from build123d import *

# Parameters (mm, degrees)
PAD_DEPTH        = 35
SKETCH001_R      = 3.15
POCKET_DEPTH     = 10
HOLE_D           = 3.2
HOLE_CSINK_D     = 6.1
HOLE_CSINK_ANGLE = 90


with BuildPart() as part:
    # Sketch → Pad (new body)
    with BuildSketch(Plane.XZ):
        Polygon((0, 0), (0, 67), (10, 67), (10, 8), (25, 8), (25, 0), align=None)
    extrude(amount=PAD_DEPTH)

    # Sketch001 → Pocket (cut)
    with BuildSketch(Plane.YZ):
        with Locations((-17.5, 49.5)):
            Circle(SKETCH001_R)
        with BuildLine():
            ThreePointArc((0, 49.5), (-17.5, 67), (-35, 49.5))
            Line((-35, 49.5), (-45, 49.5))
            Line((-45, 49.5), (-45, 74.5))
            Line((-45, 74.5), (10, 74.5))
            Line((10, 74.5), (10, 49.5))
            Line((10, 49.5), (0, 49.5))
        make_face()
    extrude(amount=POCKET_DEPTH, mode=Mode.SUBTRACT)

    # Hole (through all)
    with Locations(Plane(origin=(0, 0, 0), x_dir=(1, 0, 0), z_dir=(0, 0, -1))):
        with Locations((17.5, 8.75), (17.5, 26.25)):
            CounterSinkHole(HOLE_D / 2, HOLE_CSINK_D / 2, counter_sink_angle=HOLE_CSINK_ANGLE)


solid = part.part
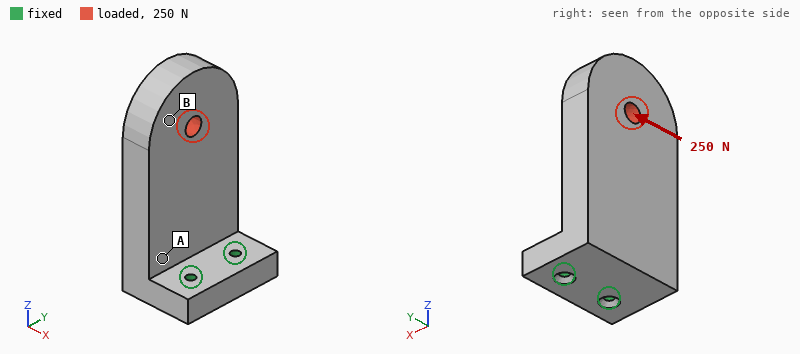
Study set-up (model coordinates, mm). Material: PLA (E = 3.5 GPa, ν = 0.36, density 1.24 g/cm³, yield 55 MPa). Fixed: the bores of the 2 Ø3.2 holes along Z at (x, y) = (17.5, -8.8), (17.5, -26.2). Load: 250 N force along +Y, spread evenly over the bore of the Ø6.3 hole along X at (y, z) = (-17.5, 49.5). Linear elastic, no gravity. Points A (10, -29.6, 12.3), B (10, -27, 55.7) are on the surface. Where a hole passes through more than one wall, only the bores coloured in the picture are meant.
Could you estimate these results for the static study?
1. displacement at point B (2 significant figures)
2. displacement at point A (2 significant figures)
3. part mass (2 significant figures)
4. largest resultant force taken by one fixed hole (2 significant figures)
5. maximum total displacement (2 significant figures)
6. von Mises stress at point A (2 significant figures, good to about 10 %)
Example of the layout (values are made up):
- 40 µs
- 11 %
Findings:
- 0.56 mm
- 0.13 mm
- 32 g
- 530 N
- 0.66 mm
- 8.8 MPa
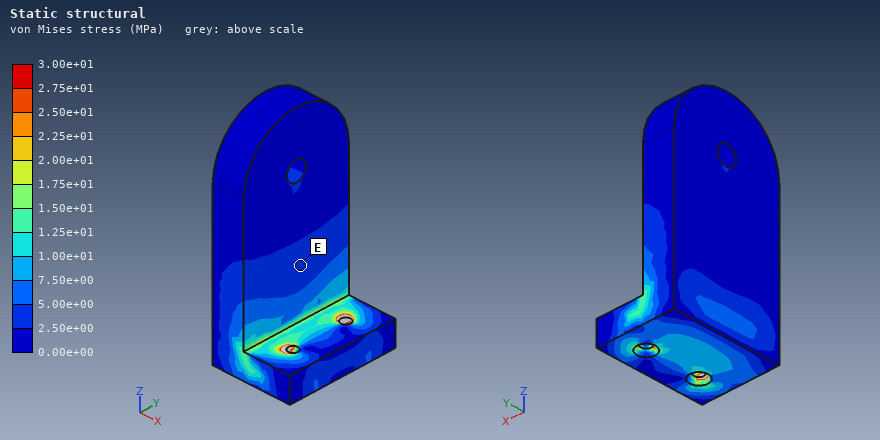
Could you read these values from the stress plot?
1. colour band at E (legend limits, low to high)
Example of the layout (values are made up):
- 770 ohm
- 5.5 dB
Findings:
- 2.50e+00 to 5.00e+00 MPa
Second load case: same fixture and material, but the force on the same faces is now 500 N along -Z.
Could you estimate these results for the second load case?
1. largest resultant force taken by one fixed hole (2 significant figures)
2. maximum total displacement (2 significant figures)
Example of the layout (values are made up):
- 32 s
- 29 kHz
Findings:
- 250 N
- 0.76 mm
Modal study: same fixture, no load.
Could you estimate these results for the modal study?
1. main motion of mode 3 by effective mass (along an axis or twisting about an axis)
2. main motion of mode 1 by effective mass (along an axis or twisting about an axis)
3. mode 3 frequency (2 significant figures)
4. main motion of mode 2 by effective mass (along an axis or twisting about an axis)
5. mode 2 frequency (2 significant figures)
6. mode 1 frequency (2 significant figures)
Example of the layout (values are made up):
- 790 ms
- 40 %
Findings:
- twisting about Z
- along X
- 2400 Hz
- along Y
- 940 Hz
- 460 Hz
